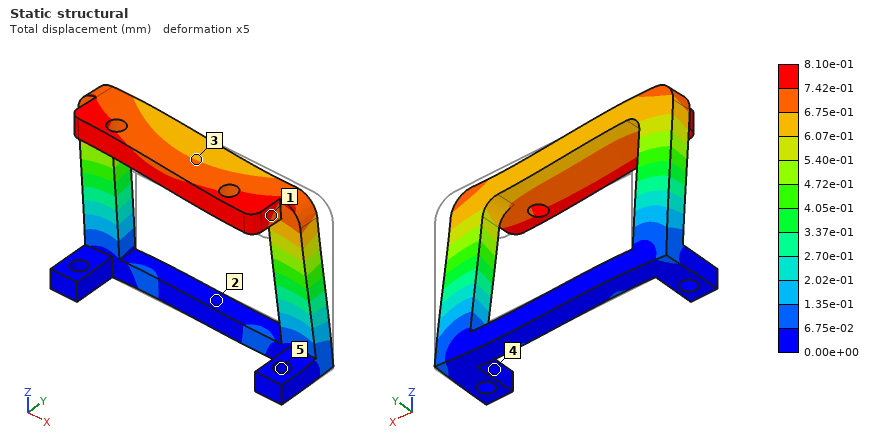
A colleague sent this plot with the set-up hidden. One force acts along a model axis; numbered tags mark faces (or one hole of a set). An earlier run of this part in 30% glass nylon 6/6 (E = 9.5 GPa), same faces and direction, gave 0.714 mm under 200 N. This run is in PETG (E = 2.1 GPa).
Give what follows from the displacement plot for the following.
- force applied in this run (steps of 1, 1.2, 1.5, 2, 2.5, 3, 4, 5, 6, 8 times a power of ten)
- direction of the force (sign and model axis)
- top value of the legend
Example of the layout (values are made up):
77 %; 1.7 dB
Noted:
50 N; -X; 8.10e-01 mm
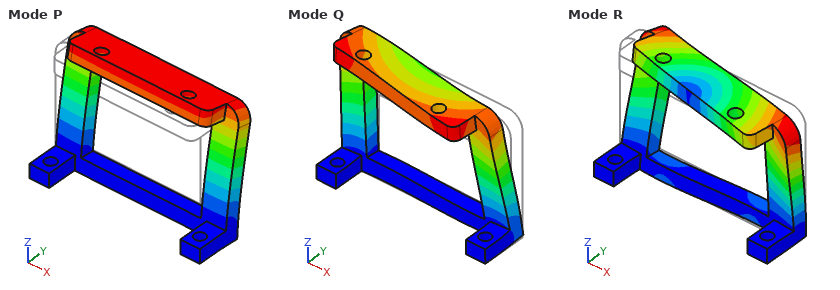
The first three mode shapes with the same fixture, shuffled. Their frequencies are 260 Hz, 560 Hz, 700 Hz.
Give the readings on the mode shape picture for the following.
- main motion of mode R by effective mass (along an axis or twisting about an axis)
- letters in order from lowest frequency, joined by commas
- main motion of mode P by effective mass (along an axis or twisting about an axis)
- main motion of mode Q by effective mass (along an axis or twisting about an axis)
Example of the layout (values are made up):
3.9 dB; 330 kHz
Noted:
along X; P, Q, R; along Y; along X
